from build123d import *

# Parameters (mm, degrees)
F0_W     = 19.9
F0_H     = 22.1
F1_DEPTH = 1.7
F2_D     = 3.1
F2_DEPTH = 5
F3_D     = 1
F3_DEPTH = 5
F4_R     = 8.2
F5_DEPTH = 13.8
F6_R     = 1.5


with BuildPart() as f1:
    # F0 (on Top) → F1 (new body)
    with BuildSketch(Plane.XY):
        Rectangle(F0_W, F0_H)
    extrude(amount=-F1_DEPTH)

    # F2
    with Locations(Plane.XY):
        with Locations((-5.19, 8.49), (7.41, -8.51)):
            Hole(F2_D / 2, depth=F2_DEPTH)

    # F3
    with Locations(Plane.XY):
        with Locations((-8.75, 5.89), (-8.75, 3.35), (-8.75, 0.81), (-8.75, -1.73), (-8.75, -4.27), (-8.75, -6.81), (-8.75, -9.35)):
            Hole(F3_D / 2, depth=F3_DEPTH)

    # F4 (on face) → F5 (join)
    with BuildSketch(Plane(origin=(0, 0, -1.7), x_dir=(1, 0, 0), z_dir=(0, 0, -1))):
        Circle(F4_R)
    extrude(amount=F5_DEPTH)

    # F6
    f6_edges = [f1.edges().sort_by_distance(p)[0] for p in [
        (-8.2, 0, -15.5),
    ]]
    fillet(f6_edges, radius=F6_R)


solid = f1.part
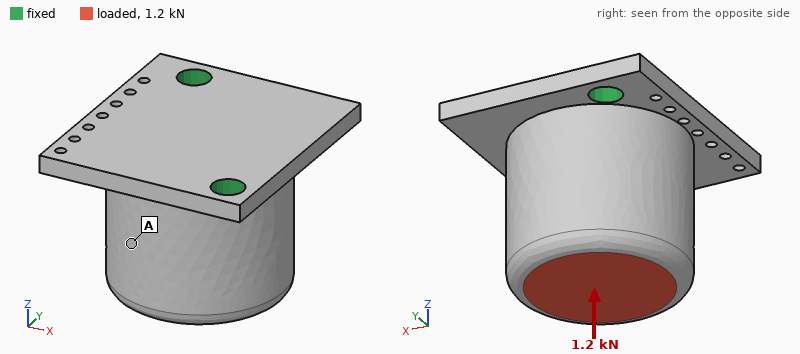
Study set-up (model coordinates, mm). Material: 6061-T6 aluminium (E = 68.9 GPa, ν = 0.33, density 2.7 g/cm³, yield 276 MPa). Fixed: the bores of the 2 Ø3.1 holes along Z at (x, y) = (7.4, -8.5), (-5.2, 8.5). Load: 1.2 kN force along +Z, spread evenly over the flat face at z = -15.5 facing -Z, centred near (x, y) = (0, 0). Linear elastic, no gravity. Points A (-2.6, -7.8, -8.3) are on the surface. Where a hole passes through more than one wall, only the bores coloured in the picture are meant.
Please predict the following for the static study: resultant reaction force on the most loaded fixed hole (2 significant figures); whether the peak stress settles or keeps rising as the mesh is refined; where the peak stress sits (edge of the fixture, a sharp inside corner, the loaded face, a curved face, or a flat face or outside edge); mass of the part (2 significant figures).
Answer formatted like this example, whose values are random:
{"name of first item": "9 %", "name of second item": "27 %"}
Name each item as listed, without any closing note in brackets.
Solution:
{"resultant reaction force on the most loaded fixed hole": "690 N", "whether the peak stress settles or keeps rising as the mesh is refined": "keeps rising", "where the peak stress sits": "edge of the fixture", "mass of the part": "9.7 g"}
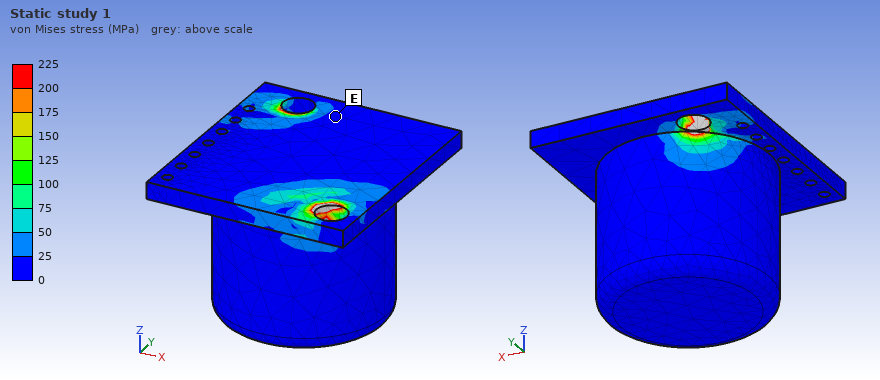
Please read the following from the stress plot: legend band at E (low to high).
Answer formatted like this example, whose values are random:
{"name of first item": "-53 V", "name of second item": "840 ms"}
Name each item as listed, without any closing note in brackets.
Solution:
{"legend band at E": "0 to 25 MPa"}
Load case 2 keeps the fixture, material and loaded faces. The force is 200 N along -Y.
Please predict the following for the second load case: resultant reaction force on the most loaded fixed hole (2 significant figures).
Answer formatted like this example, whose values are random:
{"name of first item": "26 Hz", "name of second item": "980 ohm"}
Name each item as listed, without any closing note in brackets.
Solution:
{"resultant reaction force on the most loaded fixed hole": "180 N"}
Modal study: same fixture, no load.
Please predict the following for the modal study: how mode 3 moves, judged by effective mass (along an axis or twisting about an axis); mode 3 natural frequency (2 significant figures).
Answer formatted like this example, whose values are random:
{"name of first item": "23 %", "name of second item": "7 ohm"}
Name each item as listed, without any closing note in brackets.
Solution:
{"how mode 3 moves, judged by effective mass": "along Z", "mode 3 natural frequency": "21 kHz"}
